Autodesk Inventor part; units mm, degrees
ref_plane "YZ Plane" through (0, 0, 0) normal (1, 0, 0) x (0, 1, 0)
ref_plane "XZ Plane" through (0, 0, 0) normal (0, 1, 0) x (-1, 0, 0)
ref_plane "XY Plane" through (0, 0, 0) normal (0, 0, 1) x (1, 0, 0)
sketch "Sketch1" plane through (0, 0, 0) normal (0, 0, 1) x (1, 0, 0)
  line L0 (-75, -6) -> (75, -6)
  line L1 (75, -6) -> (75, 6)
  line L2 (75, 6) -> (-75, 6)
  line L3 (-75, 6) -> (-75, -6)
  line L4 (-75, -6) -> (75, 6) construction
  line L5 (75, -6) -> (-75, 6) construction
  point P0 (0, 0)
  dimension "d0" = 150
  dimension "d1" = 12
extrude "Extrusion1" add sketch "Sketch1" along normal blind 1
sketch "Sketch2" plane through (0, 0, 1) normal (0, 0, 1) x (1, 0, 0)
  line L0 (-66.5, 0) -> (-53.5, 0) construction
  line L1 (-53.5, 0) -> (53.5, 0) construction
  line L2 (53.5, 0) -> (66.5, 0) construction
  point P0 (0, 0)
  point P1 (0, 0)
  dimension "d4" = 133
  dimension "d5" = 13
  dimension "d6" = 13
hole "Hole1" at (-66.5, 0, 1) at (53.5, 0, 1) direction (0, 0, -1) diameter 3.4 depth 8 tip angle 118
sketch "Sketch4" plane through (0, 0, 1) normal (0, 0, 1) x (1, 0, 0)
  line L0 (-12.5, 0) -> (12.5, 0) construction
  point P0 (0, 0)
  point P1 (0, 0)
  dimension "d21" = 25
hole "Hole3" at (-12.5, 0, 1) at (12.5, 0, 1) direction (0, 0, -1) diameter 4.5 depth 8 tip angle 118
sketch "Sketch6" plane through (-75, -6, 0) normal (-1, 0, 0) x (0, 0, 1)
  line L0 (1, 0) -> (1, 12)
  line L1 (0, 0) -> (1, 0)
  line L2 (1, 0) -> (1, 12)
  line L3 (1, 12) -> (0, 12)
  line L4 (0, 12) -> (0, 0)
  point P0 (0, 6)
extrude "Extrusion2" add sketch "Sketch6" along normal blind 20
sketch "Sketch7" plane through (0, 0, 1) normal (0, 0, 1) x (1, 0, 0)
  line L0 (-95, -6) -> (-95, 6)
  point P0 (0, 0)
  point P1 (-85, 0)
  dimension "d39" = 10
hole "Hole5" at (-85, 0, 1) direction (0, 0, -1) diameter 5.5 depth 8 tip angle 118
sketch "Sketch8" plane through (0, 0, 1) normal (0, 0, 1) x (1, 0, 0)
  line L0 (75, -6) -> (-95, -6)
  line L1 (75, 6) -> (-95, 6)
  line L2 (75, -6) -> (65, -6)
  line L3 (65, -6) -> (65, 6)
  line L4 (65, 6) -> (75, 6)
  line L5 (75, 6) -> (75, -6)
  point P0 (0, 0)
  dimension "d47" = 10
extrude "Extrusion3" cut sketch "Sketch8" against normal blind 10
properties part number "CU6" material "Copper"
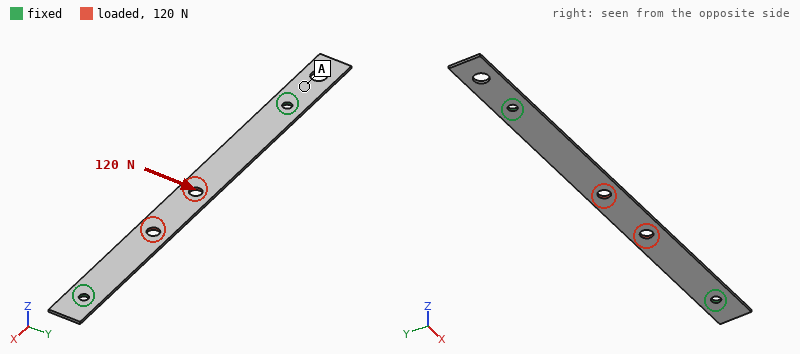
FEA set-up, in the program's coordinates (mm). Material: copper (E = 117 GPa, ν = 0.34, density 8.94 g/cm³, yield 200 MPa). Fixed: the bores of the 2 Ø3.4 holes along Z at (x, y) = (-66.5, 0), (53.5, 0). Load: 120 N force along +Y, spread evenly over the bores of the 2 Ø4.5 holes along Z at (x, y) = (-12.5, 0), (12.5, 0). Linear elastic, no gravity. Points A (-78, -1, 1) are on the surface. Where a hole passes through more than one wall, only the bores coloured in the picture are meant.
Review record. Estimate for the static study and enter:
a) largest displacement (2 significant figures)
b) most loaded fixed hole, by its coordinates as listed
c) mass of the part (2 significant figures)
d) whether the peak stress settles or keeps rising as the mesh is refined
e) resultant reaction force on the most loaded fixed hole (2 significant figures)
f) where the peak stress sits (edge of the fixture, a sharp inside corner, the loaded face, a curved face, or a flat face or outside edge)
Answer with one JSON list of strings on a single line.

["85 µm", "(53.5, 0)", "17 g", "keeps rising", "68 N", "edge of the fixture"]
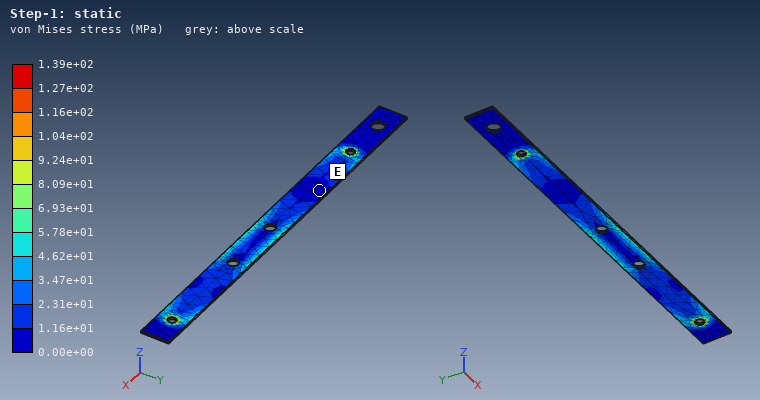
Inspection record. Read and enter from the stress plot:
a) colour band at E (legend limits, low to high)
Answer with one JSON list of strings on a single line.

["0.00e+00 to 1.16e+01 MPa"]
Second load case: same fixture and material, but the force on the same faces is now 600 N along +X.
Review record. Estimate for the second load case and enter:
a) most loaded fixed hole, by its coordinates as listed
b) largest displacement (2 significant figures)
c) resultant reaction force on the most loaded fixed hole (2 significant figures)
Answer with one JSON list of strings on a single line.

["(53.5, 0)", "12 µm", "330 N"]
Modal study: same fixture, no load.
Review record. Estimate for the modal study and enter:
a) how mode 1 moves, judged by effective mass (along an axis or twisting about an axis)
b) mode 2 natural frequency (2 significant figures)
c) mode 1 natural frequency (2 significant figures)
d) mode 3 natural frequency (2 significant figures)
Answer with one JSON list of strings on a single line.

["along Z", "740 Hz", "270 Hz", "810 Hz"]
